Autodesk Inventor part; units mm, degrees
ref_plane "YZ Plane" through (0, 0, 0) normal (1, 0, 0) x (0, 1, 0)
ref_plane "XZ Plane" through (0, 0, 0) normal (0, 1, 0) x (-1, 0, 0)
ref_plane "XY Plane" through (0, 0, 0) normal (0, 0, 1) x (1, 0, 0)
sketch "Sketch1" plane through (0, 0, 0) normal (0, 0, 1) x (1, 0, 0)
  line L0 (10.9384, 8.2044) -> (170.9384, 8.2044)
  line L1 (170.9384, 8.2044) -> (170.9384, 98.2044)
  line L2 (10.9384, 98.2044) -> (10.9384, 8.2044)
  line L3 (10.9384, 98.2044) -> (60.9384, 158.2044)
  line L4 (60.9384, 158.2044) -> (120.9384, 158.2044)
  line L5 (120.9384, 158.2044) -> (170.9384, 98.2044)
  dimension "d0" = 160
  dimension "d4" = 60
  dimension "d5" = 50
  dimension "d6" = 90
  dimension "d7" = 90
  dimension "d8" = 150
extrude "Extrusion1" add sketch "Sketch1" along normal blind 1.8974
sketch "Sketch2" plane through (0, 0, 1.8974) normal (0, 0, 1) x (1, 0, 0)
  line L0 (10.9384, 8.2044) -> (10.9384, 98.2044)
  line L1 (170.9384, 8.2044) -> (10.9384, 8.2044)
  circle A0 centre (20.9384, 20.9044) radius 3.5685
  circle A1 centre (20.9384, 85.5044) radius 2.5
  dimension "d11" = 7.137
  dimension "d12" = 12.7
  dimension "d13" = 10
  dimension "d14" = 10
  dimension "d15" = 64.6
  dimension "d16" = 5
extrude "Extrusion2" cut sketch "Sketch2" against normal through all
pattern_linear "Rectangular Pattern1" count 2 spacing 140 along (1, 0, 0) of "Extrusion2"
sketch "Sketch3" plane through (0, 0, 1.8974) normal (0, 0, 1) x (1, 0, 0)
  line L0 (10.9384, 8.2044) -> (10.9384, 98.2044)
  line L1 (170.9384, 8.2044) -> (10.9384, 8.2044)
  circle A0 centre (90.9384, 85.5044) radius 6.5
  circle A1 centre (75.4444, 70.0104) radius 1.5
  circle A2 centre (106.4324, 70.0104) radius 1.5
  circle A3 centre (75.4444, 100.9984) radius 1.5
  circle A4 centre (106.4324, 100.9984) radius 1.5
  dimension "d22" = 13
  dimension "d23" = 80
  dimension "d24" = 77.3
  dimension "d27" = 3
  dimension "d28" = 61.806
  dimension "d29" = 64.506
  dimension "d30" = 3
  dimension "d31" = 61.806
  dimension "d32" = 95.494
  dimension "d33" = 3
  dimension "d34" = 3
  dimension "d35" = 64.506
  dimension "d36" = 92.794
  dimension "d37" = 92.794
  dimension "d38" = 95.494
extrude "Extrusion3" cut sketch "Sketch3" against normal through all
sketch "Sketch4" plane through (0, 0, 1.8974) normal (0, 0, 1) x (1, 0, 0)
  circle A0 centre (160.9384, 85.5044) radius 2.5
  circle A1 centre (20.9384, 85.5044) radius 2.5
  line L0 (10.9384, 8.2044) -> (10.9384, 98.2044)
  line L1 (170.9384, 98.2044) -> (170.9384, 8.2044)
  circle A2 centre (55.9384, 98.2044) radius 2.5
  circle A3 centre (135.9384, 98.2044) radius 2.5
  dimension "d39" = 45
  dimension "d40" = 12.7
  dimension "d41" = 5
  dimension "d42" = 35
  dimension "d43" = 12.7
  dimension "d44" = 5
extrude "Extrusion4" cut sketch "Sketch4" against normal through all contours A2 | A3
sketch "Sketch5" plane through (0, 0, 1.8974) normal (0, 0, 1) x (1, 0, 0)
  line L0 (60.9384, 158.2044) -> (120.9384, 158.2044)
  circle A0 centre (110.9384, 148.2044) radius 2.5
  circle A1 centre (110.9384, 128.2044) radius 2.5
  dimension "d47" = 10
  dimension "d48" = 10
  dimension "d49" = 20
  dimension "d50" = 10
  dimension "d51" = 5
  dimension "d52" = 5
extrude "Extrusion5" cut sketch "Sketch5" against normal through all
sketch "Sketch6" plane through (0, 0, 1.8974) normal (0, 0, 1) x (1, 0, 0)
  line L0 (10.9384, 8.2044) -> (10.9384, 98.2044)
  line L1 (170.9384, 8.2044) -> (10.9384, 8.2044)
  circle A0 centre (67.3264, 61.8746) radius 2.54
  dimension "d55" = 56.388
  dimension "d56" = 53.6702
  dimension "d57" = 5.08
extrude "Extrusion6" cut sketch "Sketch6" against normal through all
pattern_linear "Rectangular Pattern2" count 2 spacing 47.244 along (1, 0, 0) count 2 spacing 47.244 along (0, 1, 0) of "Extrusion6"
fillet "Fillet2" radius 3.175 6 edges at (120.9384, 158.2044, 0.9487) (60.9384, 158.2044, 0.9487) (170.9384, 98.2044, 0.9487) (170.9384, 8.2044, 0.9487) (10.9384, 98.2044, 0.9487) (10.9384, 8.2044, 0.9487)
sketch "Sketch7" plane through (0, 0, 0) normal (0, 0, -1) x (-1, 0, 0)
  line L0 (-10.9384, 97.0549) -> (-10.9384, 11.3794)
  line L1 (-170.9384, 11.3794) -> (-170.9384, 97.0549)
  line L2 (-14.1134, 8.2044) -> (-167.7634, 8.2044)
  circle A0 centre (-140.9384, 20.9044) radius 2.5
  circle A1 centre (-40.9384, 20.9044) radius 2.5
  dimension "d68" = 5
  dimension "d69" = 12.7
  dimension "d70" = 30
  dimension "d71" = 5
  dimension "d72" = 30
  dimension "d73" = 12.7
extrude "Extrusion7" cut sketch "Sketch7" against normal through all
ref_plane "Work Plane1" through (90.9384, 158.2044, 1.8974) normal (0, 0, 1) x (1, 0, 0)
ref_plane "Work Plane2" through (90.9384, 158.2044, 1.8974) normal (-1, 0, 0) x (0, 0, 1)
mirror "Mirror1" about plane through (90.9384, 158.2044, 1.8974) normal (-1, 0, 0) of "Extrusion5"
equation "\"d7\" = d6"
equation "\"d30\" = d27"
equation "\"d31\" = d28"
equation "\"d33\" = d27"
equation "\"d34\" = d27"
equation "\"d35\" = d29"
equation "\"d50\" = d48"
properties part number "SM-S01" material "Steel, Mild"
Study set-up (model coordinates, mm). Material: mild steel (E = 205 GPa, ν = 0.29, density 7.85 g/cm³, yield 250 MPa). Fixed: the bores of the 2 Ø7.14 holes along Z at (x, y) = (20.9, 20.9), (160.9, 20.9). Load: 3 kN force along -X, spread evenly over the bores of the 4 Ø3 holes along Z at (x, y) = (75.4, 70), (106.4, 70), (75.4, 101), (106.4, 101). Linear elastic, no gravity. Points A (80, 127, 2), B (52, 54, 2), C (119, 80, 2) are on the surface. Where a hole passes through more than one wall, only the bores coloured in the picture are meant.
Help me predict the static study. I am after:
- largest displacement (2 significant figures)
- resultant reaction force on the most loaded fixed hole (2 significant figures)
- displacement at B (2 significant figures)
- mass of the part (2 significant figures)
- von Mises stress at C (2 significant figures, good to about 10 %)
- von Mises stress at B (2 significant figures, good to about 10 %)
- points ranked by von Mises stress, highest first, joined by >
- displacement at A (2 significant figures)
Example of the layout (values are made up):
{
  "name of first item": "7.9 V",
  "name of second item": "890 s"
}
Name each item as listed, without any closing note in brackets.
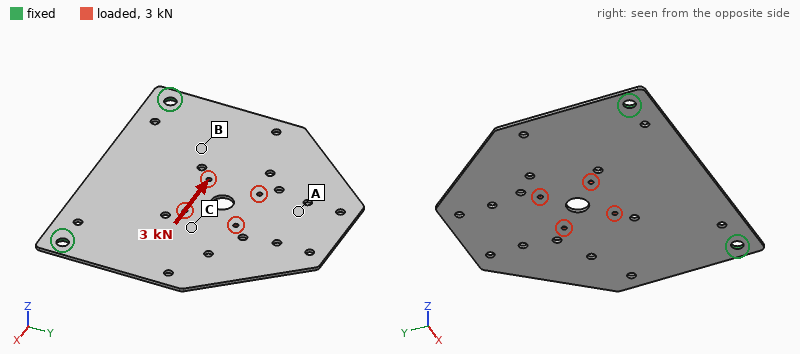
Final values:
{
  "largest displacement": "19 µm",
  "resultant reaction force on the most loaded fixed hole": "2.0 kN",
  "displacement at B": "8.2 µm",
  "mass of the part": "300 g",
  "von Mises stress at C": "13 MPa",
  "von Mises stress at B": "21 MPa",
  "points ranked by von Mises stress, highest first, joined by >": "B > C > A",
  "displacement at A": "17 µm"
}
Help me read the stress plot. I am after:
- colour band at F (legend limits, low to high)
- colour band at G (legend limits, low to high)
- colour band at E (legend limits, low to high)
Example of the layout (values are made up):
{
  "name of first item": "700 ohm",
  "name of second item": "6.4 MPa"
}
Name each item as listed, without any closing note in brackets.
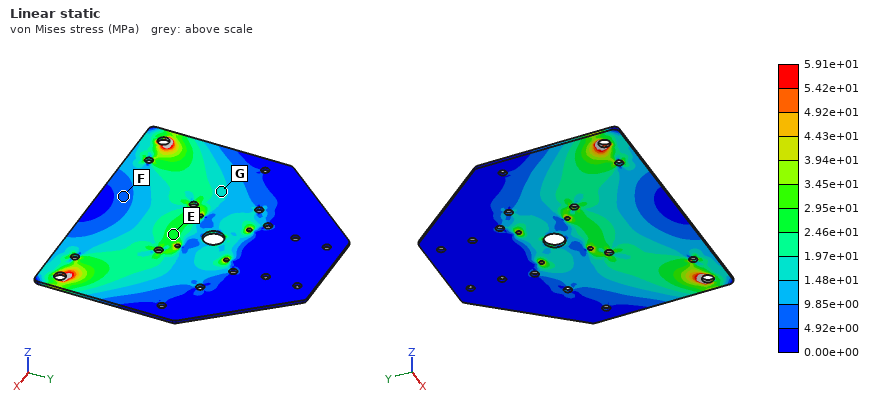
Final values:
{
  "colour band at F": "4.92e+00 to 9.85e+00 MPa",
  "colour band at G": "1.48e+01 to 1.97e+01 MPa",
  "colour band at E": "2.46e+01 to 2.95e+01 MPa"
}
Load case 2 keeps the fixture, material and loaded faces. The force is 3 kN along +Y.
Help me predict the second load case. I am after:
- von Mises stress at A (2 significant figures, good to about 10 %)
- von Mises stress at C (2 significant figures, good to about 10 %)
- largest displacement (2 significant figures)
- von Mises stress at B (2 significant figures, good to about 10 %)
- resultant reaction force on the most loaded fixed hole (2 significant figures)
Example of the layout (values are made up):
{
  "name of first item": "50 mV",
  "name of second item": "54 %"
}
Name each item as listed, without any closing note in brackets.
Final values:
{
  "von Mises stress at A": "7.8 MPa",
  "von Mises stress at C": "16 MPa",
  "largest displacement": "11 µm",
  "von Mises stress at B": "16 MPa",
  "resultant reaction force on the most loaded fixed hole": "1.6 kN"
}
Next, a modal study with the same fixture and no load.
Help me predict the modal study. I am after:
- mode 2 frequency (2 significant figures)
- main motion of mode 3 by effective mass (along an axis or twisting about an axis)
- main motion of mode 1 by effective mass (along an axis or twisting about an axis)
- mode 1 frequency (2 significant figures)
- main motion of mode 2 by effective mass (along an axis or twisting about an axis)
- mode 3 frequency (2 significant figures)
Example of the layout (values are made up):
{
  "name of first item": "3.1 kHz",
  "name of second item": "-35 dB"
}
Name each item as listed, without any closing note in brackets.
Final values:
{
  "mode 2 frequency": "270 Hz",
  "main motion of mode 3 by effective mass": "along Z",
  "main motion of mode 1 by effective mass": "along Z",
  "mode 1 frequency": "83 Hz",
  "main motion of mode 2 by effective mass": "twisting about Y",
  "mode 3 frequency": "440 Hz"
}
